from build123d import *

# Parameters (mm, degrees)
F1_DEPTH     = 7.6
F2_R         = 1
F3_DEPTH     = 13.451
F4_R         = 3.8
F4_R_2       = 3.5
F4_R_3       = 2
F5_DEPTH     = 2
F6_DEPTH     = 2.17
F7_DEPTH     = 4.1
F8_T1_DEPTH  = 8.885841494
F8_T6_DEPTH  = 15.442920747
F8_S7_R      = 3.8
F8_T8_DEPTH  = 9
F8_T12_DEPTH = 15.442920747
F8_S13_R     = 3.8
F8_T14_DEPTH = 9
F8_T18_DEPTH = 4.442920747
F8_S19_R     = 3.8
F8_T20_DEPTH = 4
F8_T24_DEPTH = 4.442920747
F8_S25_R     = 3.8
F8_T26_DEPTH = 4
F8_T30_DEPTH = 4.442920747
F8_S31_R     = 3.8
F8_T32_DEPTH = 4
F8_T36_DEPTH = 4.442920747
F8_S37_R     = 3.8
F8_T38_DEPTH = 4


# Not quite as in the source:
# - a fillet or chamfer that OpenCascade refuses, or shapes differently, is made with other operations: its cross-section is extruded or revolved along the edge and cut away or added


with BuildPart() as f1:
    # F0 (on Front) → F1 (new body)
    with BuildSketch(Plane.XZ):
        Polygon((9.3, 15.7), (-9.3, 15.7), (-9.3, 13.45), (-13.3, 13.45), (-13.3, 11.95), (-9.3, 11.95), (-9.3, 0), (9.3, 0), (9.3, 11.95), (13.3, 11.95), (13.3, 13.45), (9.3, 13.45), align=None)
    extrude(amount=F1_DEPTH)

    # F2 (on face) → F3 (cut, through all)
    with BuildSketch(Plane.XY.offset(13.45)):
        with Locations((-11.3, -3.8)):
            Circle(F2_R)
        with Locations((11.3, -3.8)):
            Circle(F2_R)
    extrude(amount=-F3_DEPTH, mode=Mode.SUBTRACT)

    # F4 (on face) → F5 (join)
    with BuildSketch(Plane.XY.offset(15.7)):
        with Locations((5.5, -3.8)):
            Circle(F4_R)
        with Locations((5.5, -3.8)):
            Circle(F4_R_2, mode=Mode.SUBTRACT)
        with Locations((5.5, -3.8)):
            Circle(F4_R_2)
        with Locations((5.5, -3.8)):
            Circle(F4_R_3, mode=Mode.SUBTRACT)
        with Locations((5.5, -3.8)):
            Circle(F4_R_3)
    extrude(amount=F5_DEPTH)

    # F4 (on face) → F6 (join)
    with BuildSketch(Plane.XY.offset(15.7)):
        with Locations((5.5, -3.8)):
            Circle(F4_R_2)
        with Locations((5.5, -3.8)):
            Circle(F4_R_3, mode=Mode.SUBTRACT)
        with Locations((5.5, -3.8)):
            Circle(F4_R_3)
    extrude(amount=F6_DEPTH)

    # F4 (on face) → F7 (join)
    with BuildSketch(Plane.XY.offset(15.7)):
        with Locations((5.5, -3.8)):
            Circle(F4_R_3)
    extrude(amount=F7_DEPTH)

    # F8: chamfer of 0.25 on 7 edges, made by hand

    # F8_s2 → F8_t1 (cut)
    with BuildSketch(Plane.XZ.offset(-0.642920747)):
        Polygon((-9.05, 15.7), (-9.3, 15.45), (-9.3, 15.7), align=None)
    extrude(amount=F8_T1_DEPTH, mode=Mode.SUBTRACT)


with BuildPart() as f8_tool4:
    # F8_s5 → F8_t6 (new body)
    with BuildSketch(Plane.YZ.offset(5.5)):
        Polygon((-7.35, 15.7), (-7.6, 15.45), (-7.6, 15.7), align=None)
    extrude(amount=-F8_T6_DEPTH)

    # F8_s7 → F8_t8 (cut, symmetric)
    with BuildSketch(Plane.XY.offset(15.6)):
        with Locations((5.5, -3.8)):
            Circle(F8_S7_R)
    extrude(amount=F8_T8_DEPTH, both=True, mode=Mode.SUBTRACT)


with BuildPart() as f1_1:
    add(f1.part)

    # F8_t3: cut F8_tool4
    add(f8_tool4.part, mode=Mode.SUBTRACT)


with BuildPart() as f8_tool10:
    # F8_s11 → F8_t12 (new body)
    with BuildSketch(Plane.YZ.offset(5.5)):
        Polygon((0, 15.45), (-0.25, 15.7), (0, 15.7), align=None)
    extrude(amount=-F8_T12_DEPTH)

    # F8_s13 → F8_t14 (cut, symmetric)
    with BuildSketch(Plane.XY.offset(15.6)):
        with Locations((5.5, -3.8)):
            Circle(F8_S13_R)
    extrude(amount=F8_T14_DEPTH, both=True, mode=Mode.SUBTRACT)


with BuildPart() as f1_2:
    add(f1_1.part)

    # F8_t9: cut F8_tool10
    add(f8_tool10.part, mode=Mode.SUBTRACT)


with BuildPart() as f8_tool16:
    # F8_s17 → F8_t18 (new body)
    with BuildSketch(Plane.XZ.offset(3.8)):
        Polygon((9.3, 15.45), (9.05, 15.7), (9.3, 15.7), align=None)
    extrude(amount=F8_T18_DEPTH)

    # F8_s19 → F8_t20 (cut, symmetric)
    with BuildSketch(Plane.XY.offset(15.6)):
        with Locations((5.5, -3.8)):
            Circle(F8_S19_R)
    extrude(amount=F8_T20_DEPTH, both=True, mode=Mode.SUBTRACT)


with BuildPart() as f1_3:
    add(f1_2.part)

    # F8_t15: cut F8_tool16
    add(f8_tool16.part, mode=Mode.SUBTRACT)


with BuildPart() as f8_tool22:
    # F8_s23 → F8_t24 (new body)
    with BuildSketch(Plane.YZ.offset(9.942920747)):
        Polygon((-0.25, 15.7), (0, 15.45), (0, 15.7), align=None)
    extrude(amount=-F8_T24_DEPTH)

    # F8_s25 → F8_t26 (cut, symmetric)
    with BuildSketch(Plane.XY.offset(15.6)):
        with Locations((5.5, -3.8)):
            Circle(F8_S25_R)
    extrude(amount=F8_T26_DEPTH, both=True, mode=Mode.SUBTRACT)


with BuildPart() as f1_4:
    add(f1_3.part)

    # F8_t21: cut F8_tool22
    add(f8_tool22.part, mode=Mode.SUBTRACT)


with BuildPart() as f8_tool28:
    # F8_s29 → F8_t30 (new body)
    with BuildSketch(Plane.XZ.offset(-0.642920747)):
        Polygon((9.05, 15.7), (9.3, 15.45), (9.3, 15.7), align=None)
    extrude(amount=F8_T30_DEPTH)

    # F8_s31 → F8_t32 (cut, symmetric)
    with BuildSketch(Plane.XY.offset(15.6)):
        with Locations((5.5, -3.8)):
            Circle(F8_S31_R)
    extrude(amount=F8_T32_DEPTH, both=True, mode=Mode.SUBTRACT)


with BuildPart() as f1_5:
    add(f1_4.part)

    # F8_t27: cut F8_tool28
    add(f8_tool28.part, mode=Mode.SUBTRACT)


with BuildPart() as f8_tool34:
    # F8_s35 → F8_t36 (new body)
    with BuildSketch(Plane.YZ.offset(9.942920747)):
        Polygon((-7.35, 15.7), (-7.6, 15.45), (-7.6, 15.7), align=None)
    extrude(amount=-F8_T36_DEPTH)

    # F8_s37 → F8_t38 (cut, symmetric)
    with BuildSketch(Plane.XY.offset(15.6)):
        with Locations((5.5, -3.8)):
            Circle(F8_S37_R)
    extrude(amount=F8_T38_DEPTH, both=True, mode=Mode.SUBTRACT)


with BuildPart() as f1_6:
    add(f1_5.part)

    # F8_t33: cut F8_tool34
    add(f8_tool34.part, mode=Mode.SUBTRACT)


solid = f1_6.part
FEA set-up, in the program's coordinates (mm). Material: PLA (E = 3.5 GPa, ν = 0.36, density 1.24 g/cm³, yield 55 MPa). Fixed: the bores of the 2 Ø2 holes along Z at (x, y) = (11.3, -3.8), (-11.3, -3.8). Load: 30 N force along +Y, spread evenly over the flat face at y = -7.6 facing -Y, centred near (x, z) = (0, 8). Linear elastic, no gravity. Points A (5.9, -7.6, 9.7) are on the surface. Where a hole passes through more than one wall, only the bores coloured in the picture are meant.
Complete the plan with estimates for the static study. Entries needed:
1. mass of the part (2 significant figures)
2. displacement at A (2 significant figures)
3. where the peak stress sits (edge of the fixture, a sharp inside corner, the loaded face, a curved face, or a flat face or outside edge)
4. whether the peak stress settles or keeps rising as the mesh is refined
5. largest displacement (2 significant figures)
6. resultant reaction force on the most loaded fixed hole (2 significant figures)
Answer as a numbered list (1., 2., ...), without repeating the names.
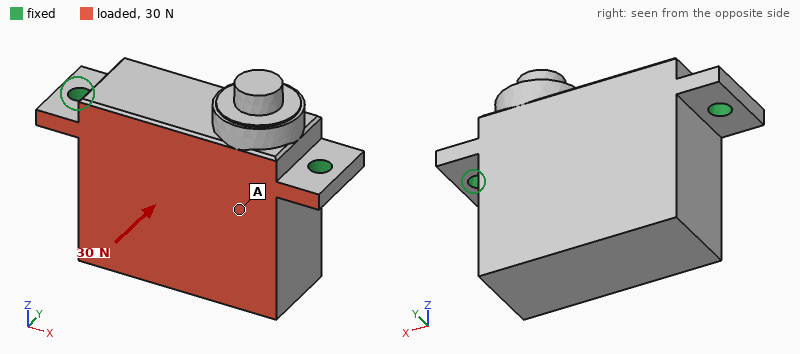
1. 3.0 g
2. 0.048 mm
3. edge of the fixture
4. keeps rising
5. 0.13 mm
6. 15 N
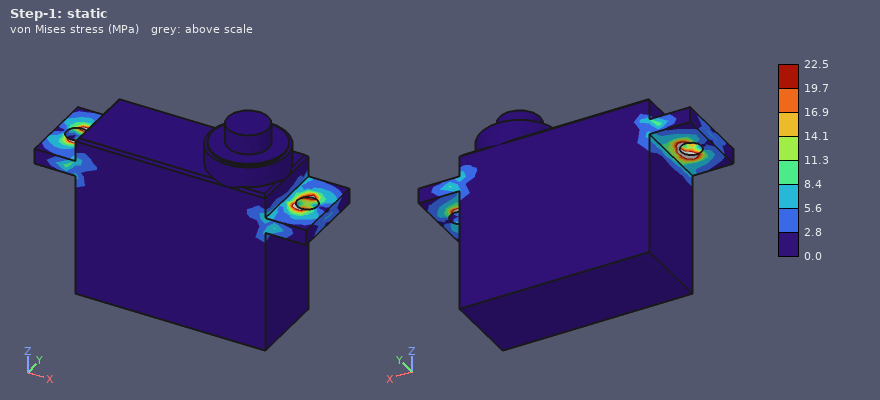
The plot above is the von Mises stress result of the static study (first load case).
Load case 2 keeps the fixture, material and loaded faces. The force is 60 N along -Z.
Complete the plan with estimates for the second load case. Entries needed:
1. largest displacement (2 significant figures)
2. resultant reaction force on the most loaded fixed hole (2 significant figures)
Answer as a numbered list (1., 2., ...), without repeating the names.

1. 0.20 mm
2. 30 N
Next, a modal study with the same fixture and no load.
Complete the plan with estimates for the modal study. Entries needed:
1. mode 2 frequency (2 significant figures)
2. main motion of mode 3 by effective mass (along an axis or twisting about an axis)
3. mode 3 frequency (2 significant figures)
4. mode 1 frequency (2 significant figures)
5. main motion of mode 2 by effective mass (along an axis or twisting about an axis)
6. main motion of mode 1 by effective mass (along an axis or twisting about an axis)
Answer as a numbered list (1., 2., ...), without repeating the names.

1. 6700 Hz
2. along X
3. 7400 Hz
4. 1700 Hz
5. along Z
6. along Y
